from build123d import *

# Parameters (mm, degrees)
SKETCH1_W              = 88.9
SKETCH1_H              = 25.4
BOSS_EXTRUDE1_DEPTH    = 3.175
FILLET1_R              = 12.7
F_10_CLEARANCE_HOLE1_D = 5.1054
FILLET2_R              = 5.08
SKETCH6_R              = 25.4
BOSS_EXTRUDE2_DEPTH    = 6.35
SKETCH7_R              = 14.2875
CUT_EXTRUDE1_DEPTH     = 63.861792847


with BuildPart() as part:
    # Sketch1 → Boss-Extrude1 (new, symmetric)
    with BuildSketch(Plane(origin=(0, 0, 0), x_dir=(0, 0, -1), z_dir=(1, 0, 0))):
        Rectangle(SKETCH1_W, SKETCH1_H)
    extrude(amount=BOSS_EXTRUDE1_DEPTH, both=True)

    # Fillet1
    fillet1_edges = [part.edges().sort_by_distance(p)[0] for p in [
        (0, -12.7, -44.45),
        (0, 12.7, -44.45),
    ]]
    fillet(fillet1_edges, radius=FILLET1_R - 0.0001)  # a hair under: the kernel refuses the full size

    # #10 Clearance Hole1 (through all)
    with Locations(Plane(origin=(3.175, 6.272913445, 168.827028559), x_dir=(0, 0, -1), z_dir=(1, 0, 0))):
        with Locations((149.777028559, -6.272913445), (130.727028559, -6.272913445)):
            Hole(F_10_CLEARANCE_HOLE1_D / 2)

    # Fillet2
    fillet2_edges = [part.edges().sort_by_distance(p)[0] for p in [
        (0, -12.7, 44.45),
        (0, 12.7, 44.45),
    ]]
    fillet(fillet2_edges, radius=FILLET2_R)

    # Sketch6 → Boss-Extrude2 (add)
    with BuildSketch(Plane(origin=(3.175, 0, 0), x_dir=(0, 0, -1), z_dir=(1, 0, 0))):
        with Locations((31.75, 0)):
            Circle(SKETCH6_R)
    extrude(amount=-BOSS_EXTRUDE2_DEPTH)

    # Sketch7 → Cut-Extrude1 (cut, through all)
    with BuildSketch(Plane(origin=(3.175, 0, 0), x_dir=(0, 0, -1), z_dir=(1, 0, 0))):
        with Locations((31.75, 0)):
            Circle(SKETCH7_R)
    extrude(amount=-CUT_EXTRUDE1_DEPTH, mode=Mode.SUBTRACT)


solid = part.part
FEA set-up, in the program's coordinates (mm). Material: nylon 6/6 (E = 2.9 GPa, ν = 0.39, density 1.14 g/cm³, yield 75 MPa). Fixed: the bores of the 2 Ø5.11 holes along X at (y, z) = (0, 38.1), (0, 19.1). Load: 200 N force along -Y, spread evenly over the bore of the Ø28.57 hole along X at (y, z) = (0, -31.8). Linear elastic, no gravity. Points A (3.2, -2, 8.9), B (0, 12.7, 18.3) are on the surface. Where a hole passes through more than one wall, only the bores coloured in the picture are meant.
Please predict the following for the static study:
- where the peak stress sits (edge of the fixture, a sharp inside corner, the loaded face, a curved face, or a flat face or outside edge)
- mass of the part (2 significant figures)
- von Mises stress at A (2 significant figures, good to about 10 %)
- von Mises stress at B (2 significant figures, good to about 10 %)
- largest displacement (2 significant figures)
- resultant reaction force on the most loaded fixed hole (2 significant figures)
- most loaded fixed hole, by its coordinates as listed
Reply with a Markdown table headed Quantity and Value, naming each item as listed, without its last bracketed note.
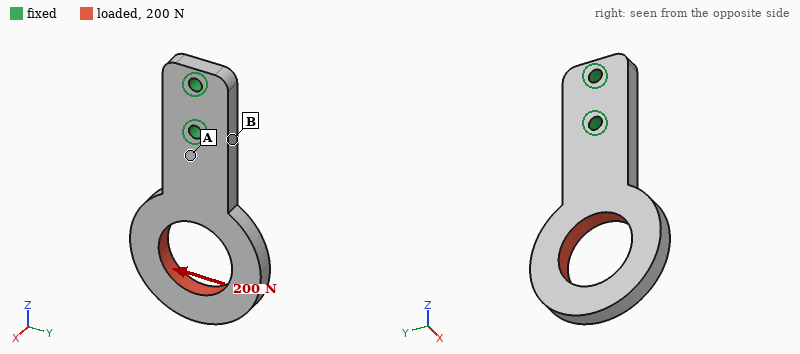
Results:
| Quantity | Value |
|---|---|
| where the peak stress sits | edge of the fixture |
| mass of the part | 19 g |
| von Mises stress at A | 3.6 MPa |
| von Mises stress at B | 14 MPa |
| largest displacement | 1.2 mm |
| resultant reaction force on the most loaded fixed hole | 560 N |
| most loaded fixed hole, by its coordinates as listed | (0, 19.1) |
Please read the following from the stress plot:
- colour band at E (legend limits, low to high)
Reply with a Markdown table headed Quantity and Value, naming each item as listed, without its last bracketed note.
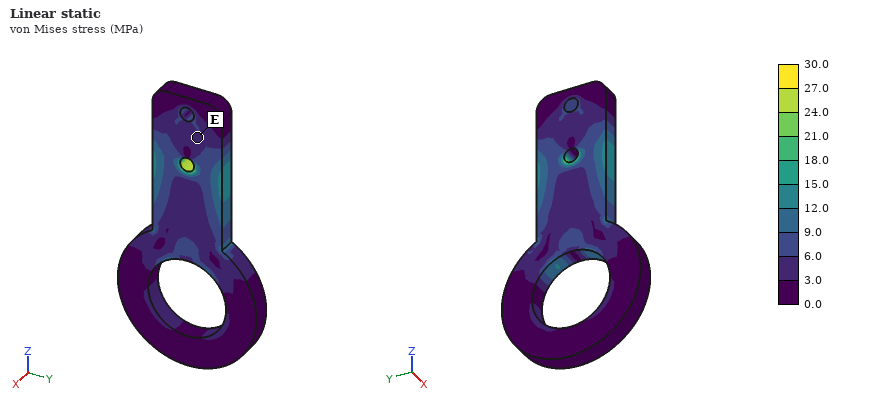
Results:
| Quantity | Value |
|---|---|
| colour band at E | 3.0 to 6.0 MPa |
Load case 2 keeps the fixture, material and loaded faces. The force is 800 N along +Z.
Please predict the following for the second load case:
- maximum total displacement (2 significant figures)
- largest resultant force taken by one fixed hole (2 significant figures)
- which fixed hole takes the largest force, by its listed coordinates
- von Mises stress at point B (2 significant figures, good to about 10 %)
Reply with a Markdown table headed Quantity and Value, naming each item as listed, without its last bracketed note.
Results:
| Quantity | Value |
|---|---|
| maximum total displacement | 0.24 mm |
| largest resultant force taken by one fixed hole | 650 N |
| which fixed hole takes the largest force, by its listed coordinates | (0, 19.1) |
| von Mises stress at point B | 2.8 MPa |
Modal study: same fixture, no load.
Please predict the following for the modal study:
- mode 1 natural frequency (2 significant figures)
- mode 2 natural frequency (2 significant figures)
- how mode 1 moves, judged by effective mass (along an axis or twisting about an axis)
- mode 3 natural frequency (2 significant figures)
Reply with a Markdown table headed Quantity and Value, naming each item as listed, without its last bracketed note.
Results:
| Quantity | Value |
|---|---|
| mode 1 natural frequency | 270 Hz |
| mode 2 natural frequency | 700 Hz |
| how mode 1 moves, judged by effective mass | along X |
| mode 3 natural frequency | 720 Hz |
